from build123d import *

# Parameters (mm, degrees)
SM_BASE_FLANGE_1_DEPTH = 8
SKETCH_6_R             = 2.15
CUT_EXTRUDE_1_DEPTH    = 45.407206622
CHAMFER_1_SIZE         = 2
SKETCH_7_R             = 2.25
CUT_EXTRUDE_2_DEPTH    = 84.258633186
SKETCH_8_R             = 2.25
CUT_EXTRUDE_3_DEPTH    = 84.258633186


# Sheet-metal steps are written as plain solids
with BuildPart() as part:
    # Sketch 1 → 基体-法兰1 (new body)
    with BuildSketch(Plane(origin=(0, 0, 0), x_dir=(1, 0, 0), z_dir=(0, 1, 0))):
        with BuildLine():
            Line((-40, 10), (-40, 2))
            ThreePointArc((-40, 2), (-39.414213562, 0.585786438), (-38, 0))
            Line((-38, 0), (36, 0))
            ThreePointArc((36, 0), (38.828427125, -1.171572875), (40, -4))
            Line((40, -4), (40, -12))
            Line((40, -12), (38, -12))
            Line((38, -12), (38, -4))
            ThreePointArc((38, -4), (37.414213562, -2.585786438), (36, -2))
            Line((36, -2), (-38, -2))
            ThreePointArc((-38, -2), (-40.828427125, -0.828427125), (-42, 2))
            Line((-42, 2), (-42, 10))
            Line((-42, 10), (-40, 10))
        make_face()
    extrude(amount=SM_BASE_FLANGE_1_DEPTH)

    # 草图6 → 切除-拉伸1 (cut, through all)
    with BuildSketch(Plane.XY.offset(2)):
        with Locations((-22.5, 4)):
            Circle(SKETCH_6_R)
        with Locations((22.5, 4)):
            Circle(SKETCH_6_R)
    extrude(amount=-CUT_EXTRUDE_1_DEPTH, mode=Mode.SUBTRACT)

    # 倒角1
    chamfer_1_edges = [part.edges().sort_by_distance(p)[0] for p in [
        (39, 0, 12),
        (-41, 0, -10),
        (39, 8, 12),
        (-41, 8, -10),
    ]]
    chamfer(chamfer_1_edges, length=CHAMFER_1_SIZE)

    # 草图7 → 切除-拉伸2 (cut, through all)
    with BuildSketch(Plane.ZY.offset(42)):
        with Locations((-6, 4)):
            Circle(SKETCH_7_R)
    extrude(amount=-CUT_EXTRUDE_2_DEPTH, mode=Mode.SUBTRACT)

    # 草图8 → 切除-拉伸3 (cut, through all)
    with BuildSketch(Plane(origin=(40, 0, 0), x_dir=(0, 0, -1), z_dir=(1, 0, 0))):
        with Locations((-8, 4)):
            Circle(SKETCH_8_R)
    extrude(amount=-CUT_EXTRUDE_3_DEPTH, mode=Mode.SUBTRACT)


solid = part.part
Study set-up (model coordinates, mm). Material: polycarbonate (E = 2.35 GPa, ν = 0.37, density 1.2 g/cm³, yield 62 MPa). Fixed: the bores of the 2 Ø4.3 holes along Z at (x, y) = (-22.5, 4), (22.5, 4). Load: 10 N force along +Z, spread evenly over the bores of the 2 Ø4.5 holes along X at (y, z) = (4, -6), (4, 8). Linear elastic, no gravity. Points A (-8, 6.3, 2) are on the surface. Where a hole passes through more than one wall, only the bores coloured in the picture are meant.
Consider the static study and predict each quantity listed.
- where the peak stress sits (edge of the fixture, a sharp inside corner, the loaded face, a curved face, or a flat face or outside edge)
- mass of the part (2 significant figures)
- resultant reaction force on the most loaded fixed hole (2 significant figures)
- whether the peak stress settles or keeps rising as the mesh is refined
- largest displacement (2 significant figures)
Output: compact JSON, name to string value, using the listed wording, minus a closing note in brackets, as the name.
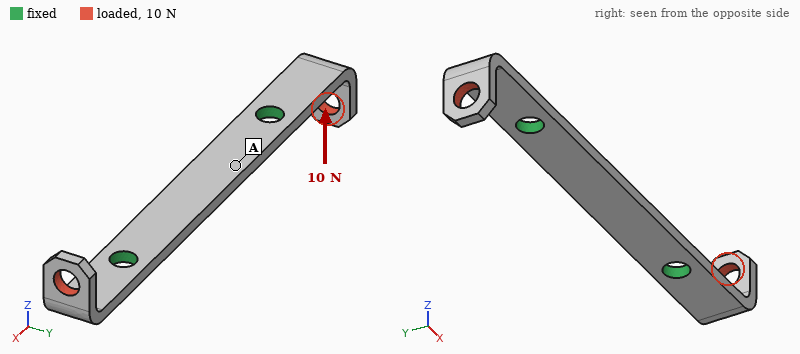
{"where the peak stress sits": "edge of the fixture", "mass of the part": "1.7 g", "resultant reaction force on the most loaded fixed hole": "5.0 N", "whether the peak stress settles or keeps rising as the mesh is refined": "keeps rising", "largest displacement": "0.91 mm"}
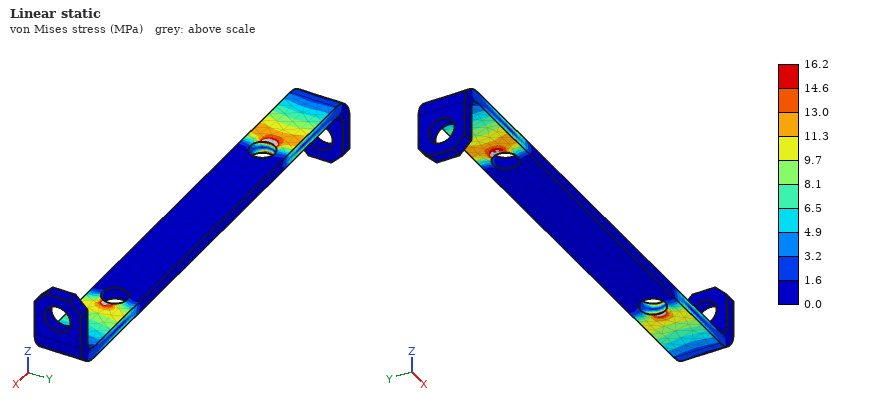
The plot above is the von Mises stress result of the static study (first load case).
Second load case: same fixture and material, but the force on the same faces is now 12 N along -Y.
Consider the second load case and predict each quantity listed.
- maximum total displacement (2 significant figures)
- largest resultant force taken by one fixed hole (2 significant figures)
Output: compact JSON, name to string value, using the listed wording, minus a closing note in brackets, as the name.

{"maximum total displacement": "0.52 mm", "largest resultant force taken by one fixed hole": "6.0 N"}
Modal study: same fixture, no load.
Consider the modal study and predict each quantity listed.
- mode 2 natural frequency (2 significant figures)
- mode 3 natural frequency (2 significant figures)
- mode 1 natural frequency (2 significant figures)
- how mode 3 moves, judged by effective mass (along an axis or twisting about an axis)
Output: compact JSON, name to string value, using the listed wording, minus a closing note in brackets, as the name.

{"mode 2 natural frequency": "1100 Hz", "mode 3 natural frequency": "1700 Hz", "mode 1 natural frequency": "880 Hz", "how mode 3 moves, judged by effective mass": "along Z"}
